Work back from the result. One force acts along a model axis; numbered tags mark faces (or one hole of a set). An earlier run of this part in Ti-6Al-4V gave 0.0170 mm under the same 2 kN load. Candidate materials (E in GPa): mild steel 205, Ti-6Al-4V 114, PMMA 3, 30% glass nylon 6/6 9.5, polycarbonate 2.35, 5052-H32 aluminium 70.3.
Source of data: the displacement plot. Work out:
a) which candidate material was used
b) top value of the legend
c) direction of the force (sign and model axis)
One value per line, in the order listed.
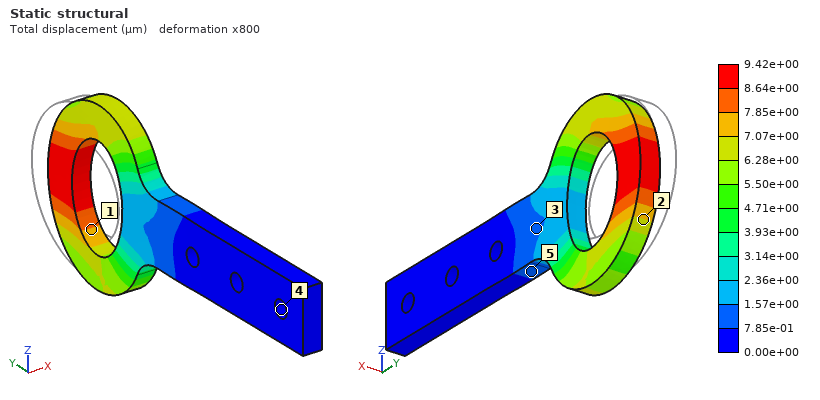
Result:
mild steel
9.42e+00 µm
-Y
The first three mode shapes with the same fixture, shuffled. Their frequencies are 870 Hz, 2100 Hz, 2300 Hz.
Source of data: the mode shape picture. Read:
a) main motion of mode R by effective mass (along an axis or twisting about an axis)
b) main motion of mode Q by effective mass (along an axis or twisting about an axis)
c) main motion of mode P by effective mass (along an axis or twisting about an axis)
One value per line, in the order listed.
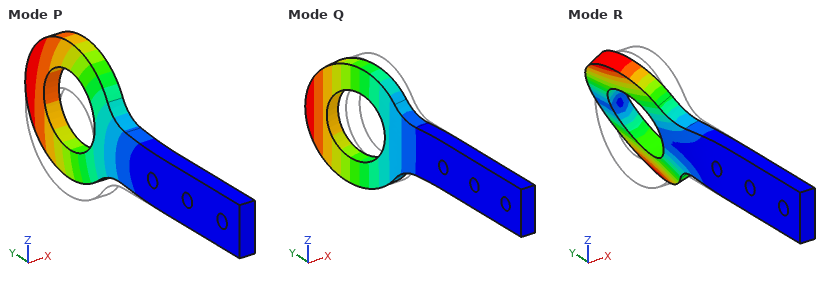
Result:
twisting about Y
along X
along Z
